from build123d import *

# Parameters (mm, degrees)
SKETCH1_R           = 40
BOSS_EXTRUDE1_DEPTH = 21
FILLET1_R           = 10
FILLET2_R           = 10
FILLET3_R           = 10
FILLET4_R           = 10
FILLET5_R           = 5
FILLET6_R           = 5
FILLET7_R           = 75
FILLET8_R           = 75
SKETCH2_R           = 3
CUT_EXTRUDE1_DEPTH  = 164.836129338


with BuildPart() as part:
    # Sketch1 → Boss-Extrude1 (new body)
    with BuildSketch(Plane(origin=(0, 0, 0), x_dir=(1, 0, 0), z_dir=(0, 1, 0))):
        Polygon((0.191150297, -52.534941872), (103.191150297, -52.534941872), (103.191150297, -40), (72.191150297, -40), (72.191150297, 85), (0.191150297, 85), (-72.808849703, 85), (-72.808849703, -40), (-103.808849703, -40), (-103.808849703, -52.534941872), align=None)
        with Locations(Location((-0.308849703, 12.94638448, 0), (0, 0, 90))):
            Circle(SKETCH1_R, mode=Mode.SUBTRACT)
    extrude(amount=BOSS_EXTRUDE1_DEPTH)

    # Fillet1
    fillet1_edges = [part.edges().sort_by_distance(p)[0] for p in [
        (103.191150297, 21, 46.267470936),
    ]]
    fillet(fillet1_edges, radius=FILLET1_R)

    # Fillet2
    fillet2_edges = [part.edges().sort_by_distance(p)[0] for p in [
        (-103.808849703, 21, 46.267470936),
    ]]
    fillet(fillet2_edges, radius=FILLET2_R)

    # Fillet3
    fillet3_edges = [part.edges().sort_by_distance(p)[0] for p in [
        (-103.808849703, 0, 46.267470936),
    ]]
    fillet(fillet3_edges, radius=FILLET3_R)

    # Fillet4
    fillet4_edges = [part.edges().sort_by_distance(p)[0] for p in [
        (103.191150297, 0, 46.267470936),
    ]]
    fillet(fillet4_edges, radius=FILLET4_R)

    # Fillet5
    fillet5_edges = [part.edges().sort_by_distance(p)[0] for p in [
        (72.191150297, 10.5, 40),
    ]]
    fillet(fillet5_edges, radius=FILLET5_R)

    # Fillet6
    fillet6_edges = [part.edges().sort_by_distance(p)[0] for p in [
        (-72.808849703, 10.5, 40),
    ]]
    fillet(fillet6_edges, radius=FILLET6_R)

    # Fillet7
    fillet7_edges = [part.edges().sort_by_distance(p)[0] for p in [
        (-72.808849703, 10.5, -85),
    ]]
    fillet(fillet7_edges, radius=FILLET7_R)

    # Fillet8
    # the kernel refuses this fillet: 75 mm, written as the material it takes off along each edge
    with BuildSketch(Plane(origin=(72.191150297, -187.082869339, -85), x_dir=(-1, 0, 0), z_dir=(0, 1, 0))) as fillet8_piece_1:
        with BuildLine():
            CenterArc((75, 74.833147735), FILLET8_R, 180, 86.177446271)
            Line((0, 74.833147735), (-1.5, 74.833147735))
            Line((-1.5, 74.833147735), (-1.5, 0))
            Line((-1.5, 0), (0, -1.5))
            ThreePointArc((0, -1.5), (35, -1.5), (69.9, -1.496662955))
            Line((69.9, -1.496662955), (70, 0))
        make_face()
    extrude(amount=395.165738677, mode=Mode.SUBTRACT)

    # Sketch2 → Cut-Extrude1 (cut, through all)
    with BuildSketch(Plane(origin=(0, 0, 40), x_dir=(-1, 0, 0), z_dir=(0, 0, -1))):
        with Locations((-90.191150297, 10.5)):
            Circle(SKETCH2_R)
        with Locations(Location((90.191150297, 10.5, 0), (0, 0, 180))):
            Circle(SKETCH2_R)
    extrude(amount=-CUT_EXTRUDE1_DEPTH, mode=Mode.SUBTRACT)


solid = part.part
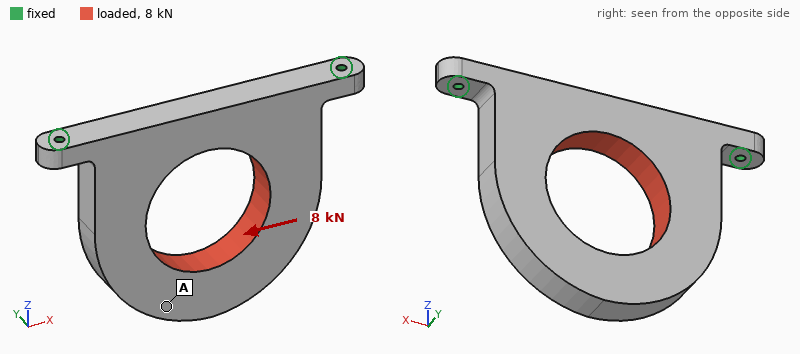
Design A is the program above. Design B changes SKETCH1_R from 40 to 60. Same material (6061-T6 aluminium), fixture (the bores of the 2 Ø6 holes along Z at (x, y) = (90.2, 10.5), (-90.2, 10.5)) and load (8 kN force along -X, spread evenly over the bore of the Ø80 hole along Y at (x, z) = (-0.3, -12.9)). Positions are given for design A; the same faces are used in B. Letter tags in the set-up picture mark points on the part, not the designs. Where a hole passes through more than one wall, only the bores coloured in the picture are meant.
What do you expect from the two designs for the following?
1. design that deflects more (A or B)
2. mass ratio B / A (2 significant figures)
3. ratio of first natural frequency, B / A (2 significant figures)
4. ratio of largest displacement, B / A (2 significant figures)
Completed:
B
0.52
1.3
9.3
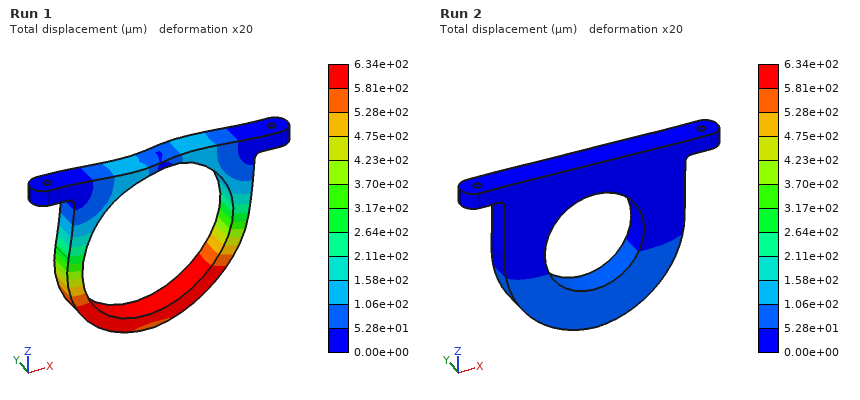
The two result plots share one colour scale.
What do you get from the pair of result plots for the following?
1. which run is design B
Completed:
Run 1
